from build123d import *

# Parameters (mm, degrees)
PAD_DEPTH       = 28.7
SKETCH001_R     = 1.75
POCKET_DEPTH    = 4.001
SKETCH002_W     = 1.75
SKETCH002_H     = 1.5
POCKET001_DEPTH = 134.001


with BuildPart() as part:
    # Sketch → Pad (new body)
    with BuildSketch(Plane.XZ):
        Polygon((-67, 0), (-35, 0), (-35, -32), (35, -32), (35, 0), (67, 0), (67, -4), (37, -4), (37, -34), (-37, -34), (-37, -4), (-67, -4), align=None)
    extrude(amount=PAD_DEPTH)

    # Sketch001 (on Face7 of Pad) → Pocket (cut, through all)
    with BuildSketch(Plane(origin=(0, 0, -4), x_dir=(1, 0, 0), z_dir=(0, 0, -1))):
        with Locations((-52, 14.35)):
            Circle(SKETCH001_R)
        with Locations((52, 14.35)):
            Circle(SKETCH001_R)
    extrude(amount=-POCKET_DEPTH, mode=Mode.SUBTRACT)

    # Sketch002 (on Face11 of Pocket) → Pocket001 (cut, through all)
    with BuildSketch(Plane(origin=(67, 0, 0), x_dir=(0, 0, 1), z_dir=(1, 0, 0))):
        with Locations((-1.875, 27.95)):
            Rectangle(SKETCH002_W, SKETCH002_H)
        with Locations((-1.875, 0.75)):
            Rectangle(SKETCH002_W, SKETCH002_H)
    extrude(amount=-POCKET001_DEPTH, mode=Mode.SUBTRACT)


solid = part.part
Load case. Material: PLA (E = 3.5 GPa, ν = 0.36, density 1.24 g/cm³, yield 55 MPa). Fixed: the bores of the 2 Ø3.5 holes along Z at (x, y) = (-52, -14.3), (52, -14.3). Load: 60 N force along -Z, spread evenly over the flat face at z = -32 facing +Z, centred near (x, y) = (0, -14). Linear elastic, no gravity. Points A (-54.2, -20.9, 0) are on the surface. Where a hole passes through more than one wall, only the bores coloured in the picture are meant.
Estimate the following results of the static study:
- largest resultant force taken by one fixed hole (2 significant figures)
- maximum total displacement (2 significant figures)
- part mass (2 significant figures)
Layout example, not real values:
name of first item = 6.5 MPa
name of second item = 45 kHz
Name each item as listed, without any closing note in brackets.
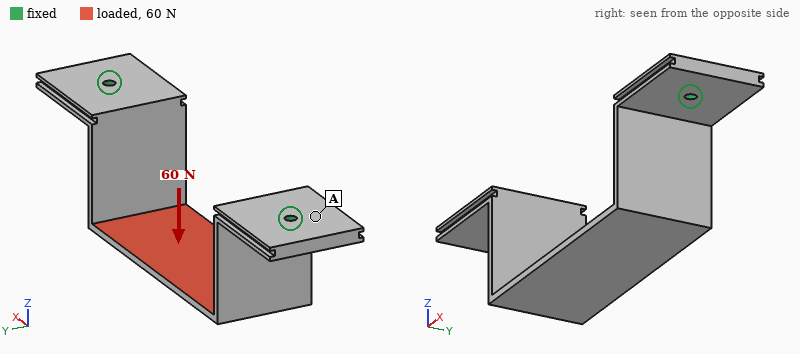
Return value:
largest resultant force taken by one fixed hole = 34 N
maximum total displacement = 1.4 mm
part mass = 18 g
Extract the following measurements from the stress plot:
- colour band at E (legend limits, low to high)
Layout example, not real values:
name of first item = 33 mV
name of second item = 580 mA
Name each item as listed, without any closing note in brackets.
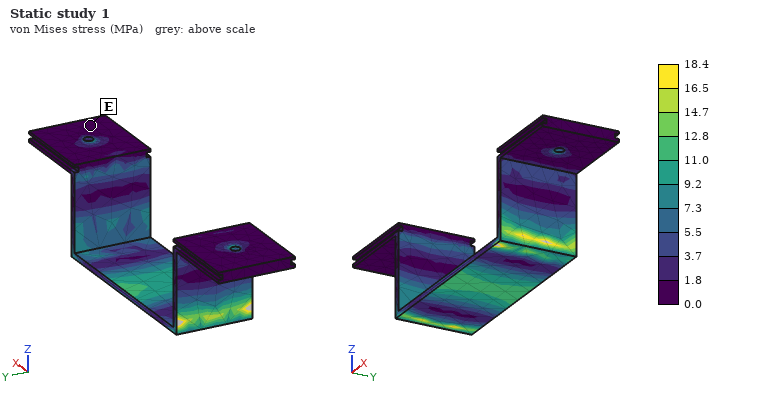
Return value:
colour band at E = 0.0 to 1.8 MPa
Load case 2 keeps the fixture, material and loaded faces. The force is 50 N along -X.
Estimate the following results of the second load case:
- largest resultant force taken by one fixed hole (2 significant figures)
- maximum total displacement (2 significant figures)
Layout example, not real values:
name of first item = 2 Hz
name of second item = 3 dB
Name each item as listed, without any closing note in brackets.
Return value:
largest resultant force taken by one fixed hole = 26 N
maximum total displacement = 1.7 mm
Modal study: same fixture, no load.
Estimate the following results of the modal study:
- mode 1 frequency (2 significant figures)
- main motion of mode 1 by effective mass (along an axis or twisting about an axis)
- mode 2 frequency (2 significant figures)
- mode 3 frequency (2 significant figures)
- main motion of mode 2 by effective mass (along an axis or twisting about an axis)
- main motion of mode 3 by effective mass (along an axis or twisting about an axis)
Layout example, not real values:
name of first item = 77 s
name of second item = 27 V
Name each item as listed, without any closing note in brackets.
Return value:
mode 1 frequency = 350 Hz
main motion of mode 1 by effective mass = along X
mode 2 frequency = 520 Hz
mode 3 frequency = 540 Hz
main motion of mode 2 by effective mass = along Y
main motion of mode 3 by effective mass = along Z
